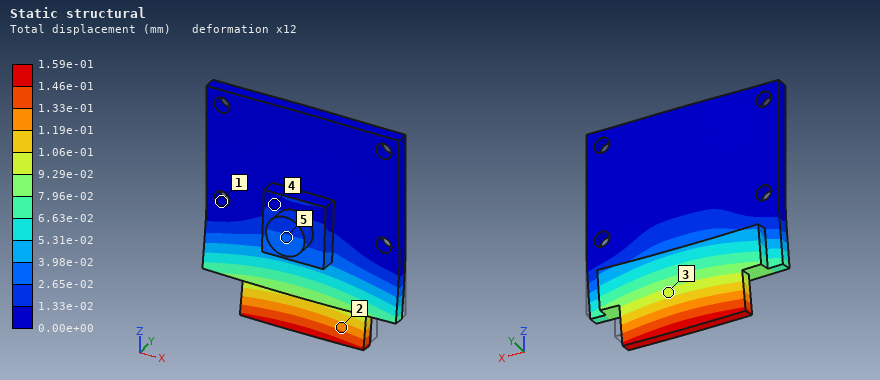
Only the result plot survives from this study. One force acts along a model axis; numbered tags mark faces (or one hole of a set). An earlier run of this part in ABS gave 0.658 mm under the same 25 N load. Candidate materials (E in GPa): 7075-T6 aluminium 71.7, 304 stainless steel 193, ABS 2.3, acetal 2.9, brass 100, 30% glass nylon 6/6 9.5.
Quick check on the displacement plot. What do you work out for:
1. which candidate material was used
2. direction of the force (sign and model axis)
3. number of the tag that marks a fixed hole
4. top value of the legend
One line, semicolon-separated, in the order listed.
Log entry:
30% glass nylon 6/6; -Y; 1; 1.59e-01 mm
